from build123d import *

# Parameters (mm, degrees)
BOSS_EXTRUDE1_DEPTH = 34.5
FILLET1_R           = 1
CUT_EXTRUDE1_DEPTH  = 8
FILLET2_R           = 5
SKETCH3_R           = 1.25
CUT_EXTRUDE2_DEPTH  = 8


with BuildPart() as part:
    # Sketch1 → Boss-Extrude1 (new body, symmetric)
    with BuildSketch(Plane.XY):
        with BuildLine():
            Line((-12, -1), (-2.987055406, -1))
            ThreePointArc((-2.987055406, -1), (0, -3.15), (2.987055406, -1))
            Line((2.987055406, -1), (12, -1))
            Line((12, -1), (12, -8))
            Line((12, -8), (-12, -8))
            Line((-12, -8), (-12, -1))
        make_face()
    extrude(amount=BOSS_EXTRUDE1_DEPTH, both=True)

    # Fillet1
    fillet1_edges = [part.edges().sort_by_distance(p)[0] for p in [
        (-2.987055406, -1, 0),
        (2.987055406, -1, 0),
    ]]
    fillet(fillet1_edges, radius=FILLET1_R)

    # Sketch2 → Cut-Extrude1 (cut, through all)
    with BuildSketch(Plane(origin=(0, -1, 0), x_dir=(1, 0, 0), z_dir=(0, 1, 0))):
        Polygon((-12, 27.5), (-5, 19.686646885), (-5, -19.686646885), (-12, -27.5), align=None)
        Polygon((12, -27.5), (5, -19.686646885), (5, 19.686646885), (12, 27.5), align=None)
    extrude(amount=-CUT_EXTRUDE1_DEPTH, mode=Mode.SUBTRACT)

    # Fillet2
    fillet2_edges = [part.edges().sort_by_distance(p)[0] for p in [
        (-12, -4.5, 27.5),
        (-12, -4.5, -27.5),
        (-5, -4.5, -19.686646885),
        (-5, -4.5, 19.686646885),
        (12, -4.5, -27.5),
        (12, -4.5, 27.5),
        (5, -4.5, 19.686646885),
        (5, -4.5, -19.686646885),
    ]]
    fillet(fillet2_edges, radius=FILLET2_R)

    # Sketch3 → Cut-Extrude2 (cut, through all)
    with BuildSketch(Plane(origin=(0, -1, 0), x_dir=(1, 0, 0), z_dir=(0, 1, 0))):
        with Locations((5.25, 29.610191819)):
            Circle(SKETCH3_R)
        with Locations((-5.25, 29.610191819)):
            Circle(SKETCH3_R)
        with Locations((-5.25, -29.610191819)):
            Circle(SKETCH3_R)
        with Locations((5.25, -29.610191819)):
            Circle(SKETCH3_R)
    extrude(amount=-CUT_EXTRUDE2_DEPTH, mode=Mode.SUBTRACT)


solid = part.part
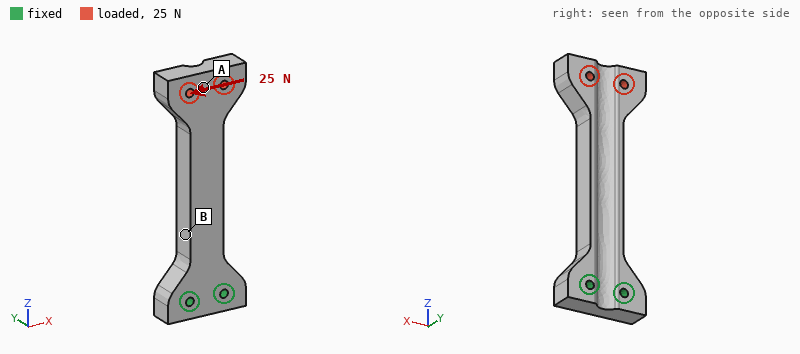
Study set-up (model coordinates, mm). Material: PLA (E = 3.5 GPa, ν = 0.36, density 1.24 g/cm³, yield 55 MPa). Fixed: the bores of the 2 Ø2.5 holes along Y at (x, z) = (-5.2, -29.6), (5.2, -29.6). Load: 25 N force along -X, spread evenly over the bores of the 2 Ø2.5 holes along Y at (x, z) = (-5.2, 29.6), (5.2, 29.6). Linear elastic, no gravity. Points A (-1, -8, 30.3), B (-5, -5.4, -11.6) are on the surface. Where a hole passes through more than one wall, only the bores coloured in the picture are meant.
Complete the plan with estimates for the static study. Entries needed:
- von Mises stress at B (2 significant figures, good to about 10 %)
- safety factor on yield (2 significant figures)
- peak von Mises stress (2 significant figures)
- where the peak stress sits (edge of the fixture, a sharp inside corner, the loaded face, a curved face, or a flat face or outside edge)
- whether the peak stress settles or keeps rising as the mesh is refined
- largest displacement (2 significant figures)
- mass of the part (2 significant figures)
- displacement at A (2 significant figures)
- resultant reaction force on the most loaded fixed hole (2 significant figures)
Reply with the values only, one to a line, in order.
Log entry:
9.2 MPa
4.1
13 MPa
a curved face
settles
0.78 mm
7.7 g
0.66 mm
130 N
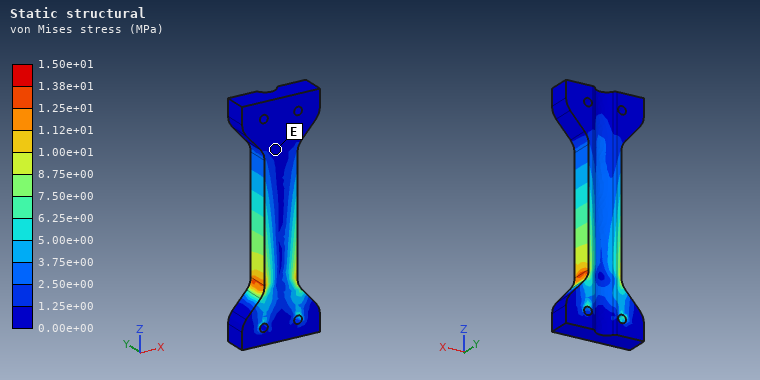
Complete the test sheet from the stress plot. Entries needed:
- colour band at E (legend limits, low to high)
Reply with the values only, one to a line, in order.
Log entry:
0.00e+00 to 1.25e+00 MPa
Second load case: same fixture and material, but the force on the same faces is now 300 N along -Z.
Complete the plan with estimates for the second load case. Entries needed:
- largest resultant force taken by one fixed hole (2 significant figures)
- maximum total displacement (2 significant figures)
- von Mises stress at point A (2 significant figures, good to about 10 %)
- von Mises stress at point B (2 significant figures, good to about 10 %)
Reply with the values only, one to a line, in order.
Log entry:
160 N
0.29 mm
1.2 MPa
4.6 MPa
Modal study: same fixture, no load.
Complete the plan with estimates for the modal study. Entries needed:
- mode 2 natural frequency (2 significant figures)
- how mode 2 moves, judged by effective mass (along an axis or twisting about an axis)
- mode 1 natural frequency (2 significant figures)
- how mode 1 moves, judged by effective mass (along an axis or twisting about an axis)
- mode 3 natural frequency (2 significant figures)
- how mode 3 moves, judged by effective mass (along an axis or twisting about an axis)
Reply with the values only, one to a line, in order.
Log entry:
600 Hz
along X
350 Hz
along Y
1500 Hz
twisting about Z
